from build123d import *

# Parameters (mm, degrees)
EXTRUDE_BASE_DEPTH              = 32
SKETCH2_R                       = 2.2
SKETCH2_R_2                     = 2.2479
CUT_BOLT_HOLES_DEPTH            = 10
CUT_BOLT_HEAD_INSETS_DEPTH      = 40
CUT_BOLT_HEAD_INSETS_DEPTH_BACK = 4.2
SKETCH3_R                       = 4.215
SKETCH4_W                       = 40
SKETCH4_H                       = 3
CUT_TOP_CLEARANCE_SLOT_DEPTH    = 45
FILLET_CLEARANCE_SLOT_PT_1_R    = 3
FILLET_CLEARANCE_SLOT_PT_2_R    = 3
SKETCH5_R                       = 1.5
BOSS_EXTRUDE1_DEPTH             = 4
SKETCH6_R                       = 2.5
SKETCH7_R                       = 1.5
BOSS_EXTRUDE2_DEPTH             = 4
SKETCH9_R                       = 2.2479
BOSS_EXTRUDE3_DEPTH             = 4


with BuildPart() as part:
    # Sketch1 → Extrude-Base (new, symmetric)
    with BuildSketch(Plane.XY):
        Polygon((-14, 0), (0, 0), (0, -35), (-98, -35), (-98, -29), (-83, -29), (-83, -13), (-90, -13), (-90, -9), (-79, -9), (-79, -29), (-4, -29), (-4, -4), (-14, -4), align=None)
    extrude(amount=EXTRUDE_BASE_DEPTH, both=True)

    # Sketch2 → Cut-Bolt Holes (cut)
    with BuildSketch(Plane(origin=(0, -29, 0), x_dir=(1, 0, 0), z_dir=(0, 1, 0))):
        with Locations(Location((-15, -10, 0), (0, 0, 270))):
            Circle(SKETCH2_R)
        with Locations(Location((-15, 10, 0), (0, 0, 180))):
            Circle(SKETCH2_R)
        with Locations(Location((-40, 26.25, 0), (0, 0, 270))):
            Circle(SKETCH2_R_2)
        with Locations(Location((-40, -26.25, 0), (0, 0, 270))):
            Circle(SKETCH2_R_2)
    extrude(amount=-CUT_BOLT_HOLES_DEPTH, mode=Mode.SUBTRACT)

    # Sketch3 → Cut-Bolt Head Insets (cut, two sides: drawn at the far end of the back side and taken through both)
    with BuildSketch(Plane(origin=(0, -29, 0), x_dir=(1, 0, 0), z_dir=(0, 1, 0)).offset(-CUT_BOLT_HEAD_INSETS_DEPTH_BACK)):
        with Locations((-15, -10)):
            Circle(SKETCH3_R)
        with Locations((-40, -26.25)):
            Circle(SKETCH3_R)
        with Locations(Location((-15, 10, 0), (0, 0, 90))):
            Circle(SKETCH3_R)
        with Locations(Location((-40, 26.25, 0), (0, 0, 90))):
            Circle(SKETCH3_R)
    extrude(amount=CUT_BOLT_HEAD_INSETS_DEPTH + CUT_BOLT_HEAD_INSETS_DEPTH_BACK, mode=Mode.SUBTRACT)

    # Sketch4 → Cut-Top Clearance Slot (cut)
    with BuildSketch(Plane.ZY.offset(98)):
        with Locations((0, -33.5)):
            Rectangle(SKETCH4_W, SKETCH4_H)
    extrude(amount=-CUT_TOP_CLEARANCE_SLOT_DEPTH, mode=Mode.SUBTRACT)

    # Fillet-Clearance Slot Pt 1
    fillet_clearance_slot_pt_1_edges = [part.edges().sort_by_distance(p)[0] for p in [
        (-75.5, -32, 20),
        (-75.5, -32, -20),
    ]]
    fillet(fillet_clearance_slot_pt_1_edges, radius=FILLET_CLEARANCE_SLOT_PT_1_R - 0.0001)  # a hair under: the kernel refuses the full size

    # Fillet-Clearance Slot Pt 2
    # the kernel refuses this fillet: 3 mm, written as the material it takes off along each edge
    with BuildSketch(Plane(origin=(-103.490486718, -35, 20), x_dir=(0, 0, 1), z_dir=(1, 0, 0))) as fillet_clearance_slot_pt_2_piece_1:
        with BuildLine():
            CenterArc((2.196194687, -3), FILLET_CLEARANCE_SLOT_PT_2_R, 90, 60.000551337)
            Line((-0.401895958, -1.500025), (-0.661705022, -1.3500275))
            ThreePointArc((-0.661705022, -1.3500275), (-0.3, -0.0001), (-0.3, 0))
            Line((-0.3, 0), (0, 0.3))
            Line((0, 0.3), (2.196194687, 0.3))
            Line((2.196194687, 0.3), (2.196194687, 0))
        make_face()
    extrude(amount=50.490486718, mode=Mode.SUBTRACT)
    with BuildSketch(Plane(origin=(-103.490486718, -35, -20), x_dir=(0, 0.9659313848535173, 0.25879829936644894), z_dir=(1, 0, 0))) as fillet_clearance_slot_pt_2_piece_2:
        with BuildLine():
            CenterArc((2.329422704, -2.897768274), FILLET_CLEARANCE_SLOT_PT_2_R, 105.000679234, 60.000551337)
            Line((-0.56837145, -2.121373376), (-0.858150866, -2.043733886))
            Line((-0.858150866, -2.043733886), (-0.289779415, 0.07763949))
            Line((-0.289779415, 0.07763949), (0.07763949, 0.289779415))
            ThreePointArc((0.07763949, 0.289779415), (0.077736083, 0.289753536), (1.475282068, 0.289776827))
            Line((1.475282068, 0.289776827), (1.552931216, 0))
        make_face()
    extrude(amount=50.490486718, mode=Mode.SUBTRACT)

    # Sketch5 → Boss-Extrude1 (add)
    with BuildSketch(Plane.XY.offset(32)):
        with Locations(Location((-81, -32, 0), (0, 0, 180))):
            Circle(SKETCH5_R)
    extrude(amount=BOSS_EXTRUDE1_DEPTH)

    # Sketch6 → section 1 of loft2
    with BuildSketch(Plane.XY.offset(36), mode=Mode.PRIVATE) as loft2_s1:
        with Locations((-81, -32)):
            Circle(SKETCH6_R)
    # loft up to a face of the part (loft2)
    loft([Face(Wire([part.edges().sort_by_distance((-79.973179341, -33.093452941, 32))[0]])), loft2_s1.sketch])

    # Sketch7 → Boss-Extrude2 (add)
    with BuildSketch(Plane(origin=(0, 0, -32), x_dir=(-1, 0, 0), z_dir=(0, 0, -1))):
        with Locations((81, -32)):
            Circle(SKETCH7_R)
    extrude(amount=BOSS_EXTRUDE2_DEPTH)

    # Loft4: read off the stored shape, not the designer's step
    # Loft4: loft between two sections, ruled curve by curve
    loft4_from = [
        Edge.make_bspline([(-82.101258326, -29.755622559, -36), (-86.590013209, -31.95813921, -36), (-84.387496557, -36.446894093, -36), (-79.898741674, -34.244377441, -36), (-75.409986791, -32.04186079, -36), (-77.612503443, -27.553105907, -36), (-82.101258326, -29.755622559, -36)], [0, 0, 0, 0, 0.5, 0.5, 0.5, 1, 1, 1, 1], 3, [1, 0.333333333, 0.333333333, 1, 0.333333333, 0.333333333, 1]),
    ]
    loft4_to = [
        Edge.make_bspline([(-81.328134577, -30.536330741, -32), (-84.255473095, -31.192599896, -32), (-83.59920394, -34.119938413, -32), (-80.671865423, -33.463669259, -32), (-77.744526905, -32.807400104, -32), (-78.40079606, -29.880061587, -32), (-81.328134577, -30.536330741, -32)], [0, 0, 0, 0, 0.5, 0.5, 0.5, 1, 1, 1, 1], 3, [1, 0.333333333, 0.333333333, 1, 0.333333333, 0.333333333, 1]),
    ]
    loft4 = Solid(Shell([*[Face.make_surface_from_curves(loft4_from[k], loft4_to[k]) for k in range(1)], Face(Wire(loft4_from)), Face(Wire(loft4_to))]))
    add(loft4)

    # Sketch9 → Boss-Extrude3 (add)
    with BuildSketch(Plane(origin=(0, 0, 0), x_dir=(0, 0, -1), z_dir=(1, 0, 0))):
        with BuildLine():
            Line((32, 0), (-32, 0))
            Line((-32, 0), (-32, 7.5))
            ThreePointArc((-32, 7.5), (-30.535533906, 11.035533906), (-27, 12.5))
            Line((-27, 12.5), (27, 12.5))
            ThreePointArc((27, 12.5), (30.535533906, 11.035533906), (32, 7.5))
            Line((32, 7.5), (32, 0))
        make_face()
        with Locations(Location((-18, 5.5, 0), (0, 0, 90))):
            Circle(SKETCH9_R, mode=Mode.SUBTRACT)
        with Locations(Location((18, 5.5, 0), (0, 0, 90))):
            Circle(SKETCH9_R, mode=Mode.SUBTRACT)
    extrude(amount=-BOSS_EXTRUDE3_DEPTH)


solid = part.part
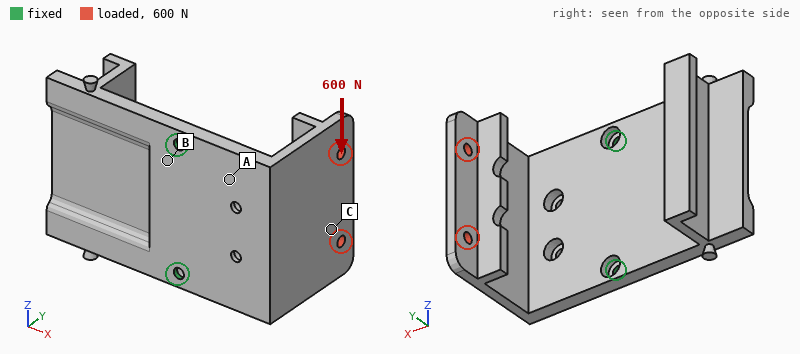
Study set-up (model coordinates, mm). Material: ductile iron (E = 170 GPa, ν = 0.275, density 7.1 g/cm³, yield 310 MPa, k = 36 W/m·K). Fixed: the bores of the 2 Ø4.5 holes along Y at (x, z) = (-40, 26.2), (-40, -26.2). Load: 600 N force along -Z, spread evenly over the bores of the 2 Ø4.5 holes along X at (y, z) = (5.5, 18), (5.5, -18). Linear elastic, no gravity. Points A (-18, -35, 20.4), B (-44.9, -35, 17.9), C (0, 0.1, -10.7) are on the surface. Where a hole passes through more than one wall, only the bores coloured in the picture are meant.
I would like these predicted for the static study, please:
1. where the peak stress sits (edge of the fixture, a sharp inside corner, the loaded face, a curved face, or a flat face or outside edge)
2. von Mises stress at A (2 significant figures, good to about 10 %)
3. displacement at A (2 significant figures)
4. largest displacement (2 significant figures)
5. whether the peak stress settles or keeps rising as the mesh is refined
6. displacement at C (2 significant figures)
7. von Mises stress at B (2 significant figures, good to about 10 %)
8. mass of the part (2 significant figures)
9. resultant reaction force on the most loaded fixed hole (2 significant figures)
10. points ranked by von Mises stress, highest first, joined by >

edge of the fixture
37 MPa
0.023 mm
0.12 mm
keeps rising
0.071 mm
12 MPa
360 g
700 N
A > B > C
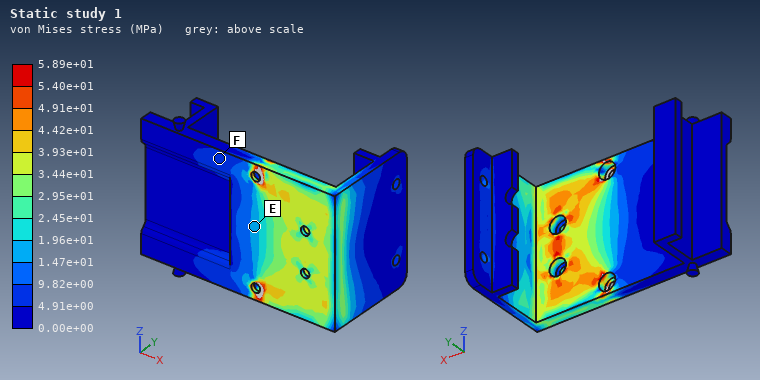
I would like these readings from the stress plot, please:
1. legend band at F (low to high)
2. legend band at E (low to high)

4.91e+00 to 9.82e+00 MPa
1.47e+01 to 1.96e+01 MPa
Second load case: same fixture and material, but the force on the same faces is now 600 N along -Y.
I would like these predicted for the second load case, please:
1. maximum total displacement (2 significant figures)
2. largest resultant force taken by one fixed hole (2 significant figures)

0.40 mm
430 N
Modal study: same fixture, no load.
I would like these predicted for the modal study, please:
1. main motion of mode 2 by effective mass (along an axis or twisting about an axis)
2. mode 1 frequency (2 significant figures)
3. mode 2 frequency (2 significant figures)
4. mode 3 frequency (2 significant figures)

along Y
460 Hz
940 Hz
1500 Hz
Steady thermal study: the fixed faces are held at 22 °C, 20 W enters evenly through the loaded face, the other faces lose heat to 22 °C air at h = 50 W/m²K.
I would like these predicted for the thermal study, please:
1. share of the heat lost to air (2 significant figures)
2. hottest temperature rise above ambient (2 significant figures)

87 %
70 K
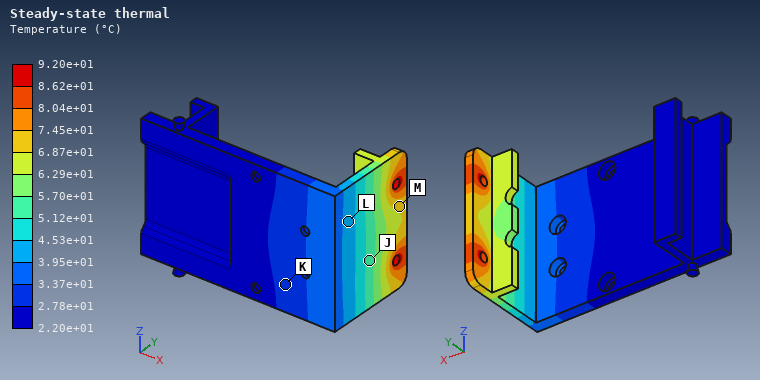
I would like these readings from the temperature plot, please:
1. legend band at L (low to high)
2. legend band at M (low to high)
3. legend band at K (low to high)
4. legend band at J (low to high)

3.95e+01 to 4.53e+01 °C
6.87e+01 to 7.45e+01 °C
2.78e+01 to 3.37e+01 °C
5.12e+01 to 5.70e+01 °C
